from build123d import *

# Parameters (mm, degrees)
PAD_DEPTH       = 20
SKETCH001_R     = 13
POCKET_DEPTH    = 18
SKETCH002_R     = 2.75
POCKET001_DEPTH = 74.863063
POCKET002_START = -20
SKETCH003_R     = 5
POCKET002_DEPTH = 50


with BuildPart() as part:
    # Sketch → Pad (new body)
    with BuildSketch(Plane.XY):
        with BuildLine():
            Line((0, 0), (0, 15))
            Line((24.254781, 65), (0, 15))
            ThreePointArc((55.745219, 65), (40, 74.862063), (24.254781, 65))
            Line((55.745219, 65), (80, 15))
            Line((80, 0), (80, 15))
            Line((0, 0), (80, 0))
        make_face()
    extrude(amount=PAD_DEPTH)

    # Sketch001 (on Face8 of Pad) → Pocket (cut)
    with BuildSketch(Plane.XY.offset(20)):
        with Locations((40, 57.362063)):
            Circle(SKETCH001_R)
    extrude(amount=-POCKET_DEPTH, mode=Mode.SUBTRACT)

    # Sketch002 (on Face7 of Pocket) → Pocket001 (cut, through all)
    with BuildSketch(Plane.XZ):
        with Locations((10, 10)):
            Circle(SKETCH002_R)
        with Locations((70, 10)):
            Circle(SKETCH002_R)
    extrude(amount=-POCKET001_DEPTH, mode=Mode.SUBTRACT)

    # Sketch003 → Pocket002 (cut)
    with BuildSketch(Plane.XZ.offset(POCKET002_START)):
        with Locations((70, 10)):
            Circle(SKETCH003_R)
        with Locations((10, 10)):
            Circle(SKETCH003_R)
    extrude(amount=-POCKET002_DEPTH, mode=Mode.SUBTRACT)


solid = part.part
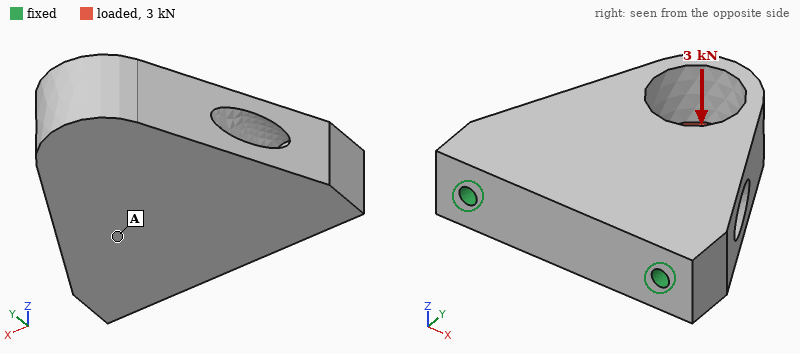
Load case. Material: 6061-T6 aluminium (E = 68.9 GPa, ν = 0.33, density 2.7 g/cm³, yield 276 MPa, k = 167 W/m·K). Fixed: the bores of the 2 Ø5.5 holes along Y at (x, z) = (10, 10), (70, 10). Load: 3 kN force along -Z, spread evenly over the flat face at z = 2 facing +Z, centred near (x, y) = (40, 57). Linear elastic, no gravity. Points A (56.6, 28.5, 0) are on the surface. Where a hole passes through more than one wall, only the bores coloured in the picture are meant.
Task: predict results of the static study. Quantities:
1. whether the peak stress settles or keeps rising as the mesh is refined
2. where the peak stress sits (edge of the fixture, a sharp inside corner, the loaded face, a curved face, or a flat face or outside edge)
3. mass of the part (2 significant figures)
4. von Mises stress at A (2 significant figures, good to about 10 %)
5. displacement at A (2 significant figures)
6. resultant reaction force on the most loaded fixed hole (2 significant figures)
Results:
keeps rising
edge of the fixture
190 g
22 MPa
0.028 mm
1.5 kN
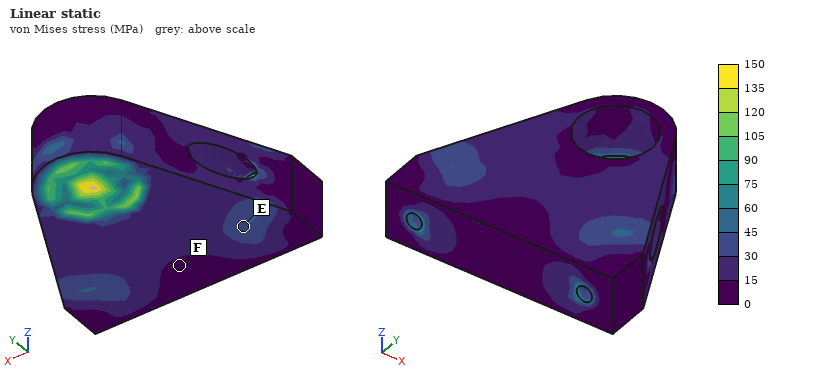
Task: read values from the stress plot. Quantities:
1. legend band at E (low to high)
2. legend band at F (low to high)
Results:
30 to 45 MPa
0 to 15 MPa
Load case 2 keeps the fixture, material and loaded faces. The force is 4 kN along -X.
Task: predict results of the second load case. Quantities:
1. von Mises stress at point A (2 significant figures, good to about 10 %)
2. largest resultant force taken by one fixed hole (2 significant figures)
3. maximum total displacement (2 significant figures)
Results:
12 MPa
3.6 kN
28 µm
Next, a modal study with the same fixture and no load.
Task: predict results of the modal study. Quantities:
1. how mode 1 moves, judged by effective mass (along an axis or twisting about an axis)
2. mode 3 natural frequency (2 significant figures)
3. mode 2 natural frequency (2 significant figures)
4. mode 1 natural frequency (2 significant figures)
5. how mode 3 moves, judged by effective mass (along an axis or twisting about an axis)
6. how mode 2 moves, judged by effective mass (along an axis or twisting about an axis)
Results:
along Z
12 kHz
11 kHz
4400 Hz
along X
along X
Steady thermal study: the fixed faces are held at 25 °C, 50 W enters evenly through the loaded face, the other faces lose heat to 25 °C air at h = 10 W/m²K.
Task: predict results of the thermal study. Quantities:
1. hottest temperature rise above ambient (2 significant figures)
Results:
33 K
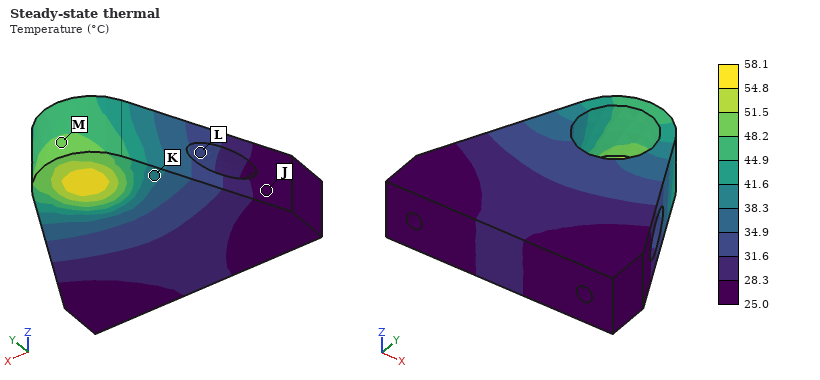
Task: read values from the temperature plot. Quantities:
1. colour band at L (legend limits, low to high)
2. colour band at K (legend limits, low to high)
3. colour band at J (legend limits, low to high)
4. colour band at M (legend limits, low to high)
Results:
31.6 to 34.9 °C
38.3 to 41.6 °C
25.0 to 28.3 °C
48.2 to 51.5 °C
